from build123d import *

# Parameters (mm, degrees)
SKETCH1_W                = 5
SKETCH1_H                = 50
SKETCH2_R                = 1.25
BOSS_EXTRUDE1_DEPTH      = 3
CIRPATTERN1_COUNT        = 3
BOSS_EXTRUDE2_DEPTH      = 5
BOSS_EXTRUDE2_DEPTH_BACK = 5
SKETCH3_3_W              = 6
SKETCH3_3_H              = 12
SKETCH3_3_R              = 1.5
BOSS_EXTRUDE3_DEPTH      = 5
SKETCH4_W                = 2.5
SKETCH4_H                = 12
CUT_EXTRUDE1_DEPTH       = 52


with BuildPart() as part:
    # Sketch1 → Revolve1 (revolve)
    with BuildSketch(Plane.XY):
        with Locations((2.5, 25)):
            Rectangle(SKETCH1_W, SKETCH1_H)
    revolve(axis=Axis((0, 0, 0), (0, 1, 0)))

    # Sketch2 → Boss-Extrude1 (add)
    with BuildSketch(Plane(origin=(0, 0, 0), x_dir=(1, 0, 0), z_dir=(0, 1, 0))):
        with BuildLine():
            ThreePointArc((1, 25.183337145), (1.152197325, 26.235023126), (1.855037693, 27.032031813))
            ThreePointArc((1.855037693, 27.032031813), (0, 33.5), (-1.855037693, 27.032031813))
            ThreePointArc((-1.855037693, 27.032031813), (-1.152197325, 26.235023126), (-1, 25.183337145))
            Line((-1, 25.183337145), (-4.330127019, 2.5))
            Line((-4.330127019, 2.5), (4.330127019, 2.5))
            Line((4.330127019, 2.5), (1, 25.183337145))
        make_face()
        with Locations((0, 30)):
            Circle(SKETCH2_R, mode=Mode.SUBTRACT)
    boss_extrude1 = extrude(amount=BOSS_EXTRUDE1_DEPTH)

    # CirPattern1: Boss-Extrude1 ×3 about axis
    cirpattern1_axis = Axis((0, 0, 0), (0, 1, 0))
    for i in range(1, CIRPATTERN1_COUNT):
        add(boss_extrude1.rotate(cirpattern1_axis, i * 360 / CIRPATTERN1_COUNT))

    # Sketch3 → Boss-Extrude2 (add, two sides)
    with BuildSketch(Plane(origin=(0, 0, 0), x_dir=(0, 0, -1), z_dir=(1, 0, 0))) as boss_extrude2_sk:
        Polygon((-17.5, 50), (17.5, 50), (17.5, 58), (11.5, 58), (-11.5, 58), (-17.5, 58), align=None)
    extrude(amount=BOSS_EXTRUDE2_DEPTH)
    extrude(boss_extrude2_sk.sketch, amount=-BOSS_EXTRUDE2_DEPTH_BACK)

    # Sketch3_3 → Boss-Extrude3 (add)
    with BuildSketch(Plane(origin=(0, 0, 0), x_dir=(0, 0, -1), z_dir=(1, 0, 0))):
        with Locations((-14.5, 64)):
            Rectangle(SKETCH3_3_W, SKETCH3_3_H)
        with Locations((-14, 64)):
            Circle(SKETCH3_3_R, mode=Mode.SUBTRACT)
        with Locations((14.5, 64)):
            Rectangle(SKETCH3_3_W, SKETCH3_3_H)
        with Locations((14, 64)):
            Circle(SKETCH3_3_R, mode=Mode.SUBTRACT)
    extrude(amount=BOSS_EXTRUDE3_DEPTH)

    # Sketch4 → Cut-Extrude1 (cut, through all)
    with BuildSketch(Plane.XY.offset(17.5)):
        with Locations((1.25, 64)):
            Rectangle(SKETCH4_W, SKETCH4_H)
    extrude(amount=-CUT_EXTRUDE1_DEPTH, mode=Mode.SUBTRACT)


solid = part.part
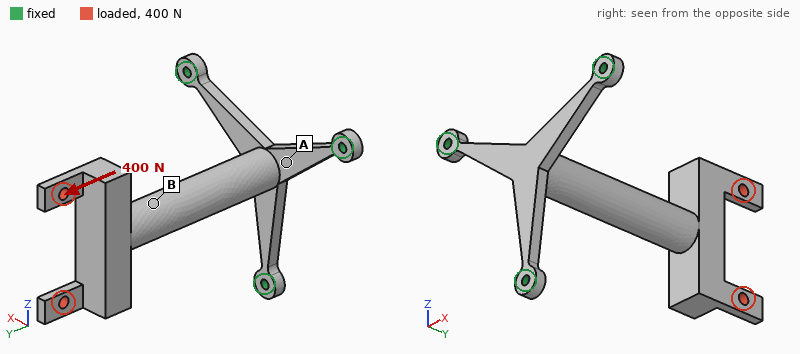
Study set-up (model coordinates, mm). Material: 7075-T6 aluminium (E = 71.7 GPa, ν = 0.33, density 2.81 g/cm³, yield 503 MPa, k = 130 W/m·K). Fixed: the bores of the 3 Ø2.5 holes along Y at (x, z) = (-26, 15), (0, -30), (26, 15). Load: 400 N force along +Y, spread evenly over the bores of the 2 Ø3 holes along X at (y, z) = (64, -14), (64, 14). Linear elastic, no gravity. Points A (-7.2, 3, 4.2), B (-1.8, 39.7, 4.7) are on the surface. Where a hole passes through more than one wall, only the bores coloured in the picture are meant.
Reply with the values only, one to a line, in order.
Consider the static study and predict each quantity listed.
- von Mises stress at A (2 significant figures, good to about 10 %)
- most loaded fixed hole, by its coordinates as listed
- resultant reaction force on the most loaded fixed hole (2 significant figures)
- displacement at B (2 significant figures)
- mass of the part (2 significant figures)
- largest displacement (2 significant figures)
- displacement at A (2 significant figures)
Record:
91 MPa
(26, 15)
170 N
0.32 mm
23 g
0.50 mm
0.21 mm
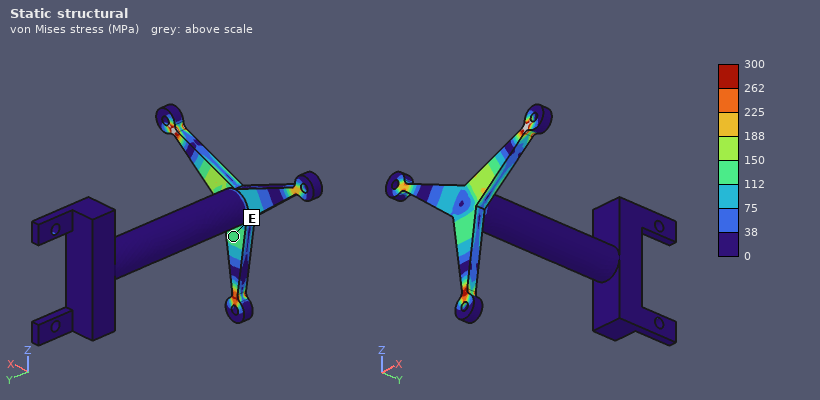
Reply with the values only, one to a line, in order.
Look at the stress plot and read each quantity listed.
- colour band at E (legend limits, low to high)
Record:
112 to 150 MPa
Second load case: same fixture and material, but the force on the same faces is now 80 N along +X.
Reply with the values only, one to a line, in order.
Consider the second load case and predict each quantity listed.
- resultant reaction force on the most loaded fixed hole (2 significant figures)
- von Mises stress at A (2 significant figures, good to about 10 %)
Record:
130 N
160 MPa
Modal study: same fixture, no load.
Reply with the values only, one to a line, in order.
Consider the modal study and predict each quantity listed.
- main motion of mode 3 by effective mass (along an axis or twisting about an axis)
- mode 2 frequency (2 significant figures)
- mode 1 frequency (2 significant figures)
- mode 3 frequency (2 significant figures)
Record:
along Y
470 Hz
470 Hz
1400 Hz
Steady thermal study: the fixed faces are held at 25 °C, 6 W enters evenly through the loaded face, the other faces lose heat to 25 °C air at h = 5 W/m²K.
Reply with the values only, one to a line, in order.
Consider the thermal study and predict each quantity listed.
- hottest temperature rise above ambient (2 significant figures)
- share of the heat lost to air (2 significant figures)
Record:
71 K
15 %
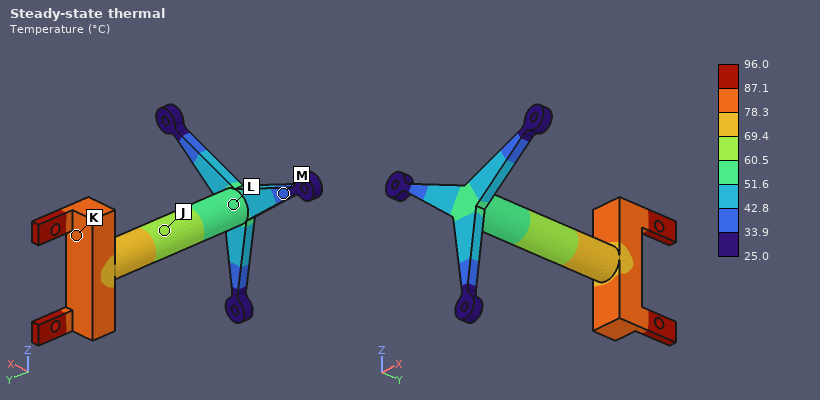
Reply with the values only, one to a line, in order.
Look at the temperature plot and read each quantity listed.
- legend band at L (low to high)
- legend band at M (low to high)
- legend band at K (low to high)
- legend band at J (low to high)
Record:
51.6 to 60.5 °C
33.9 to 42.8 °C
78.3 to 87.1 °C
60.5 to 69.4 °C
